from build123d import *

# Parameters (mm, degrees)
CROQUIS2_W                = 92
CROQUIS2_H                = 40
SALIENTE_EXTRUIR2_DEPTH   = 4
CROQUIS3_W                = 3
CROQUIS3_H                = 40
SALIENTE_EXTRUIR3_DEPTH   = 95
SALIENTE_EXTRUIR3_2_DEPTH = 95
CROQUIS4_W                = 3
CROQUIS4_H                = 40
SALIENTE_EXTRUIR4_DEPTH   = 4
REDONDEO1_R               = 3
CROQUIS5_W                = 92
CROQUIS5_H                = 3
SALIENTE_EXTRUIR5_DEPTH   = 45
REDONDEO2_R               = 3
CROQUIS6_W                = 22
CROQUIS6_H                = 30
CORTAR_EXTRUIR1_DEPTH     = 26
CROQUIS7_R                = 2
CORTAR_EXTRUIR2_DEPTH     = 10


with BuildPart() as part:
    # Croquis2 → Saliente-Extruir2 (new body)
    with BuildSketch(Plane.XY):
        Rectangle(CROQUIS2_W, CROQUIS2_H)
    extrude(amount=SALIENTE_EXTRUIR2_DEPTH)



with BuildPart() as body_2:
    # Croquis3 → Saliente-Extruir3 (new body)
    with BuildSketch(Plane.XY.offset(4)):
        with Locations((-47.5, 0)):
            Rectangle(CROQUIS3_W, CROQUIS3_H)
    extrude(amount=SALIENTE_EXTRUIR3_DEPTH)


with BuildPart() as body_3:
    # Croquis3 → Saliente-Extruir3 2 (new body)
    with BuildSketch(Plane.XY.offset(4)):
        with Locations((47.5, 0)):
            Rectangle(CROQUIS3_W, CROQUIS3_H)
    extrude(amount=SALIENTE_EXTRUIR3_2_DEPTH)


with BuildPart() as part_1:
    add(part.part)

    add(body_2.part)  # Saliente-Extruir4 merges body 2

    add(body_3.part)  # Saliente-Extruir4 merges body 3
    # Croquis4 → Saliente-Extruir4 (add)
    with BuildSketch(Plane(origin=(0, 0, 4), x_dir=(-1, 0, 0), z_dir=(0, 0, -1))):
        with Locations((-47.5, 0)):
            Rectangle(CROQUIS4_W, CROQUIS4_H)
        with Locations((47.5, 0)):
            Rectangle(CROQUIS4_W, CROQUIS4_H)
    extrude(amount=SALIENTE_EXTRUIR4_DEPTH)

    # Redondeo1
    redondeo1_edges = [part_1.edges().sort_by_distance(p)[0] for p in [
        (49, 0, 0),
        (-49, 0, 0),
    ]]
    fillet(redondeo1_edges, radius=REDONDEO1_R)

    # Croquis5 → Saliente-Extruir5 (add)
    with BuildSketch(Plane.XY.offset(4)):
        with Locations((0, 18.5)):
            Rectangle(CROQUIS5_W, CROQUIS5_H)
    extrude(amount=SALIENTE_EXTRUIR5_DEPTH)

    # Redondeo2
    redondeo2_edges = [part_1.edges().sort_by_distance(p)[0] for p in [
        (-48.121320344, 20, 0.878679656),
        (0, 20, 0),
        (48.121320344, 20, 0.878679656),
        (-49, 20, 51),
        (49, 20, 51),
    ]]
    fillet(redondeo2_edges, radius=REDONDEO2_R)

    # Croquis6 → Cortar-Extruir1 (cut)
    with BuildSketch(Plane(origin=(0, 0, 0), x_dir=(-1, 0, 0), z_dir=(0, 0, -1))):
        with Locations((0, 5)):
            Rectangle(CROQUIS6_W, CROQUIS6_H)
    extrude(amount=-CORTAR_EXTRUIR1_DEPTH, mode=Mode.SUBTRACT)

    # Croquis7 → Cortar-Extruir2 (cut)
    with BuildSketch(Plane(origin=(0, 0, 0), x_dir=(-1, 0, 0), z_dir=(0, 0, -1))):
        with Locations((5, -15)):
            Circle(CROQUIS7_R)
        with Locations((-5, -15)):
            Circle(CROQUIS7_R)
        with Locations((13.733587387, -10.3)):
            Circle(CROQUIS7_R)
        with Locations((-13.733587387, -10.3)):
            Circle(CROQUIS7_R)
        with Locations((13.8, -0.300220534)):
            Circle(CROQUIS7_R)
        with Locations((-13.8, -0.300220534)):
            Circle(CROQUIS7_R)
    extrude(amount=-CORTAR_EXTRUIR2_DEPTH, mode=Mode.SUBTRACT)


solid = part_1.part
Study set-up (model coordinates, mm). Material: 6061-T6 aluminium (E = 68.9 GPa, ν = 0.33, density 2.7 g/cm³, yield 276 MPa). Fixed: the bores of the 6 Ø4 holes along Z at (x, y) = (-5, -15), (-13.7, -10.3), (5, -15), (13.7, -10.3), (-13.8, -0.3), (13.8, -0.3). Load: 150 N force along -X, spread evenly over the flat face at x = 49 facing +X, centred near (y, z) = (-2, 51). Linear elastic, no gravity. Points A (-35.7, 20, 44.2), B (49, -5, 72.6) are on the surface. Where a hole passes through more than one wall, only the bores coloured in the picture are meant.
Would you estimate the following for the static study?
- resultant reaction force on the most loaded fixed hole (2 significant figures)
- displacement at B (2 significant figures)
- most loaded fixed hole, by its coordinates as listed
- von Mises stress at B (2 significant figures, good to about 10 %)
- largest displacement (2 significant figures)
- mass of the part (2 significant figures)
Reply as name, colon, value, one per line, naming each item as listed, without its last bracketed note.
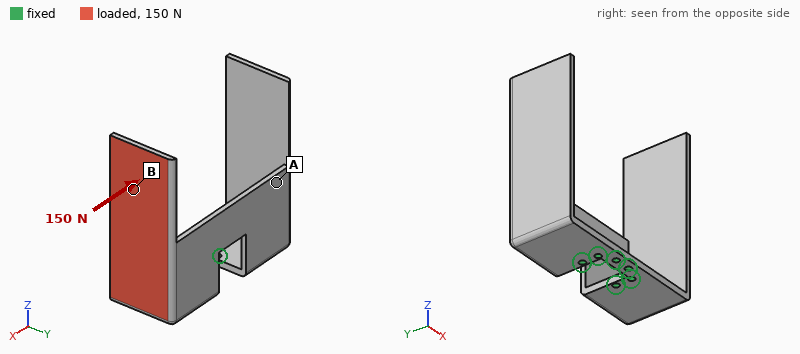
resultant reaction force on the most loaded fixed hole: 260 N
displacement at B: 0.56 mm
most loaded fixed hole, by its coordinates as listed: (-13.8, -0.3)
von Mises stress at B: 11 MPa
largest displacement: 1.0 mm
mass of the part: 120 g
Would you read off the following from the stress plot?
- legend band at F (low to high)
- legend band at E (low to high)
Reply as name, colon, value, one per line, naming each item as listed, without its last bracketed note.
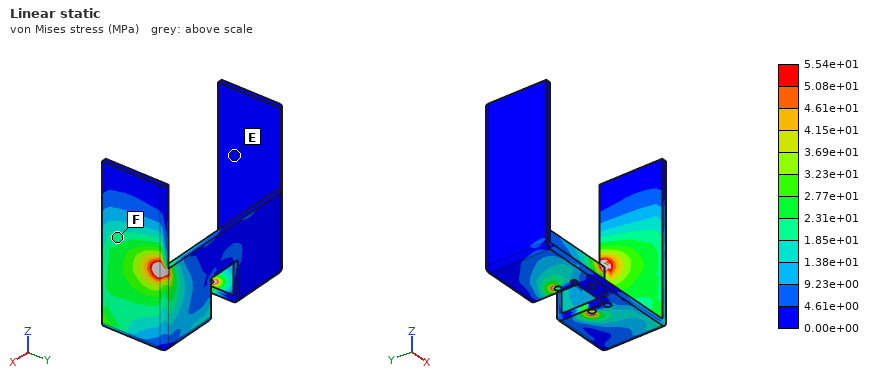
legend band at F: 1.85e+01 to 2.31e+01 MPa
legend band at E: 0.00e+00 to 4.61e+00 MPa
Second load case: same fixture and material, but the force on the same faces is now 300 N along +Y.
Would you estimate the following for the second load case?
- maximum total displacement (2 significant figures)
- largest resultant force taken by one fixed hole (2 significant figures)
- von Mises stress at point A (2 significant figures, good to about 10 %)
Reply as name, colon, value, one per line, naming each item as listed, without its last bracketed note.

maximum total displacement: 1.4 mm
largest resultant force taken by one fixed hole: 970 N
von Mises stress at point A: 21 MPa
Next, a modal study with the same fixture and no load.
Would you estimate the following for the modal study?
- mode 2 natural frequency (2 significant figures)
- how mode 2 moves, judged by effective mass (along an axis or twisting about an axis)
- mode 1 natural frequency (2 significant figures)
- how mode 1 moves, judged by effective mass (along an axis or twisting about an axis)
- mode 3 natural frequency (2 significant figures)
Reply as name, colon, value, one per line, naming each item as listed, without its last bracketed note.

mode 2 natural frequency: 460 Hz
how mode 2 moves, judged by effective mass: along Y
mode 1 natural frequency: 380 Hz
how mode 1 moves, judged by effective mass: along X
mode 3 natural frequency: 540 Hz
